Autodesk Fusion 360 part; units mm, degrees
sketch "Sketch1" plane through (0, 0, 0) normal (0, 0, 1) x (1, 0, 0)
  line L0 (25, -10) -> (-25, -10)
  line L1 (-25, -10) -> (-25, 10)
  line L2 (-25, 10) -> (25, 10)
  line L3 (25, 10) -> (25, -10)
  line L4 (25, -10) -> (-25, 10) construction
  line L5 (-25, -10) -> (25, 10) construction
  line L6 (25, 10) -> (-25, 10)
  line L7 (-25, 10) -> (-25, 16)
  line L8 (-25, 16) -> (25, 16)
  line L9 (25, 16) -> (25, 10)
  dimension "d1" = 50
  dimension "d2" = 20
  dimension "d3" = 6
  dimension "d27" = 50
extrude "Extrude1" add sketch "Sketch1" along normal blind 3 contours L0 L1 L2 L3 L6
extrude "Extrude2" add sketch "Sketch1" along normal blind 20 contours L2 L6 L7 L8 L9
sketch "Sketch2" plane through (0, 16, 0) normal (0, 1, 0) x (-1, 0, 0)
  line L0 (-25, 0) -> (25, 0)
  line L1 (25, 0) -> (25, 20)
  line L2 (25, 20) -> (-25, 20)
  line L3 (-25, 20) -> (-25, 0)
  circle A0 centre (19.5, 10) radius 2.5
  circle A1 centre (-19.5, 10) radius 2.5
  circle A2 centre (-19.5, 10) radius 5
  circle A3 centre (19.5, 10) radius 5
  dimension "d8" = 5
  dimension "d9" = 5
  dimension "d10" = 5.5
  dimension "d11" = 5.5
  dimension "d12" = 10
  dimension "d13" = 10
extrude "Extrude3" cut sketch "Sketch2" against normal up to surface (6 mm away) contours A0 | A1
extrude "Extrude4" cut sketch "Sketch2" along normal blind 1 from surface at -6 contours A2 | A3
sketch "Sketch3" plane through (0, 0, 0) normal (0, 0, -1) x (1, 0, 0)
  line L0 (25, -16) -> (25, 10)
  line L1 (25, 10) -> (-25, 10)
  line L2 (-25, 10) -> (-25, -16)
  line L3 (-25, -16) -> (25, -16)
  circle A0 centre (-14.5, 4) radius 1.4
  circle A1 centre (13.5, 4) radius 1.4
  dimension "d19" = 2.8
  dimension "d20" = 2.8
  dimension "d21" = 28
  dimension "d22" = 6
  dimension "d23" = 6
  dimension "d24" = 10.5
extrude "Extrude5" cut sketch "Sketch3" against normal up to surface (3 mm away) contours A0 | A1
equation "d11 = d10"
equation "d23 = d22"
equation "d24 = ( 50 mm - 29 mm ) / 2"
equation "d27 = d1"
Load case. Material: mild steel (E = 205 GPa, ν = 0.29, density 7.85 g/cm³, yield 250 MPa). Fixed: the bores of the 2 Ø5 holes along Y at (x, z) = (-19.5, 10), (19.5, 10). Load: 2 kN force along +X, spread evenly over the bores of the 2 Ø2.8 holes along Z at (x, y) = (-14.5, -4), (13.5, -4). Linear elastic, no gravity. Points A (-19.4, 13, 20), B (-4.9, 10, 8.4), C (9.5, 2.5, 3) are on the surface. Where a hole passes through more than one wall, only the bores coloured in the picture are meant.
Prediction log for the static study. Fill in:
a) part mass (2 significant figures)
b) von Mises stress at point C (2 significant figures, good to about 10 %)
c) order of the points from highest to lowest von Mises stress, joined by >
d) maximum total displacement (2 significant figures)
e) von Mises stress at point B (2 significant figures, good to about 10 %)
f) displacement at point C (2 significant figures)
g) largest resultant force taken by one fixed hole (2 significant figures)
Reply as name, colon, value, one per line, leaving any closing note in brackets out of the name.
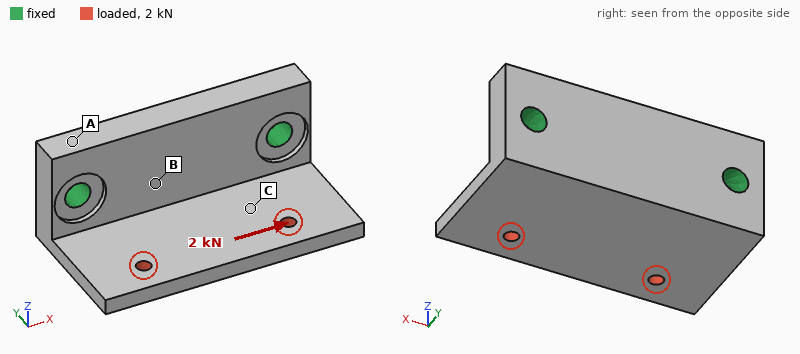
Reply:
part mass: 68 g
von Mises stress at point C: 35 MPa
order of the points from highest to lowest von Mises stress, joined by >: C > B > A
maximum total displacement: 14 µm
von Mises stress at point B: 20 MPa
displacement at point C: 5.6 µm
largest resultant force taken by one fixed hole: 1.4 kN
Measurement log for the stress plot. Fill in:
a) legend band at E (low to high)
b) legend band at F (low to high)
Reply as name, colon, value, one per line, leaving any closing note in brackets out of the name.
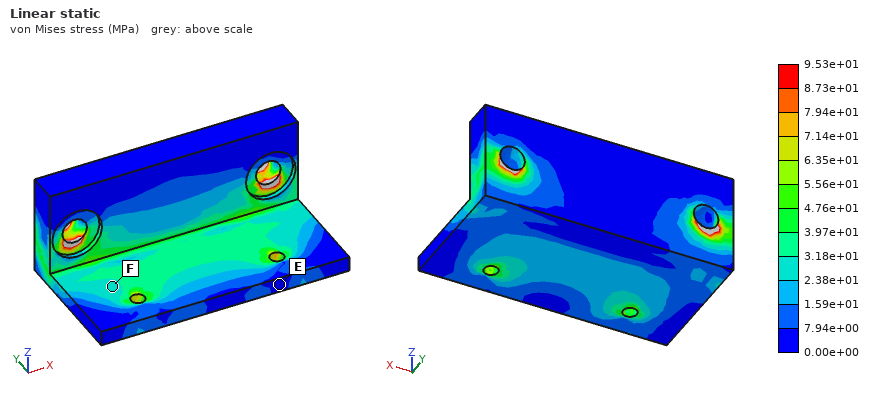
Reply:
legend band at E: 0.00e+00 to 7.94e+00 MPa
legend band at F: 2.38e+01 to 3.18e+01 MPa
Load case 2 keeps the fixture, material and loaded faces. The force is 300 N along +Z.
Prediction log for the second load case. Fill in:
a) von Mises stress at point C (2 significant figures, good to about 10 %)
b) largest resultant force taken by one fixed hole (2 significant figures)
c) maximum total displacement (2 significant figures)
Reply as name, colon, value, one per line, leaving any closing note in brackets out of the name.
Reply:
von Mises stress at point C: 25 MPa
largest resultant force taken by one fixed hole: 150 N
maximum total displacement: 33 µm
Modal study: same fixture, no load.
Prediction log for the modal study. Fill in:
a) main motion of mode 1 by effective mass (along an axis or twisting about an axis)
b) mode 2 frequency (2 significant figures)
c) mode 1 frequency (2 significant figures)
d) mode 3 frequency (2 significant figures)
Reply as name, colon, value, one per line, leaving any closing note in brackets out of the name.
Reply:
main motion of mode 1 by effective mass: along Z
mode 2 frequency: 7000 Hz
mode 1 frequency: 4700 Hz
mode 3 frequency: 12 kHz
